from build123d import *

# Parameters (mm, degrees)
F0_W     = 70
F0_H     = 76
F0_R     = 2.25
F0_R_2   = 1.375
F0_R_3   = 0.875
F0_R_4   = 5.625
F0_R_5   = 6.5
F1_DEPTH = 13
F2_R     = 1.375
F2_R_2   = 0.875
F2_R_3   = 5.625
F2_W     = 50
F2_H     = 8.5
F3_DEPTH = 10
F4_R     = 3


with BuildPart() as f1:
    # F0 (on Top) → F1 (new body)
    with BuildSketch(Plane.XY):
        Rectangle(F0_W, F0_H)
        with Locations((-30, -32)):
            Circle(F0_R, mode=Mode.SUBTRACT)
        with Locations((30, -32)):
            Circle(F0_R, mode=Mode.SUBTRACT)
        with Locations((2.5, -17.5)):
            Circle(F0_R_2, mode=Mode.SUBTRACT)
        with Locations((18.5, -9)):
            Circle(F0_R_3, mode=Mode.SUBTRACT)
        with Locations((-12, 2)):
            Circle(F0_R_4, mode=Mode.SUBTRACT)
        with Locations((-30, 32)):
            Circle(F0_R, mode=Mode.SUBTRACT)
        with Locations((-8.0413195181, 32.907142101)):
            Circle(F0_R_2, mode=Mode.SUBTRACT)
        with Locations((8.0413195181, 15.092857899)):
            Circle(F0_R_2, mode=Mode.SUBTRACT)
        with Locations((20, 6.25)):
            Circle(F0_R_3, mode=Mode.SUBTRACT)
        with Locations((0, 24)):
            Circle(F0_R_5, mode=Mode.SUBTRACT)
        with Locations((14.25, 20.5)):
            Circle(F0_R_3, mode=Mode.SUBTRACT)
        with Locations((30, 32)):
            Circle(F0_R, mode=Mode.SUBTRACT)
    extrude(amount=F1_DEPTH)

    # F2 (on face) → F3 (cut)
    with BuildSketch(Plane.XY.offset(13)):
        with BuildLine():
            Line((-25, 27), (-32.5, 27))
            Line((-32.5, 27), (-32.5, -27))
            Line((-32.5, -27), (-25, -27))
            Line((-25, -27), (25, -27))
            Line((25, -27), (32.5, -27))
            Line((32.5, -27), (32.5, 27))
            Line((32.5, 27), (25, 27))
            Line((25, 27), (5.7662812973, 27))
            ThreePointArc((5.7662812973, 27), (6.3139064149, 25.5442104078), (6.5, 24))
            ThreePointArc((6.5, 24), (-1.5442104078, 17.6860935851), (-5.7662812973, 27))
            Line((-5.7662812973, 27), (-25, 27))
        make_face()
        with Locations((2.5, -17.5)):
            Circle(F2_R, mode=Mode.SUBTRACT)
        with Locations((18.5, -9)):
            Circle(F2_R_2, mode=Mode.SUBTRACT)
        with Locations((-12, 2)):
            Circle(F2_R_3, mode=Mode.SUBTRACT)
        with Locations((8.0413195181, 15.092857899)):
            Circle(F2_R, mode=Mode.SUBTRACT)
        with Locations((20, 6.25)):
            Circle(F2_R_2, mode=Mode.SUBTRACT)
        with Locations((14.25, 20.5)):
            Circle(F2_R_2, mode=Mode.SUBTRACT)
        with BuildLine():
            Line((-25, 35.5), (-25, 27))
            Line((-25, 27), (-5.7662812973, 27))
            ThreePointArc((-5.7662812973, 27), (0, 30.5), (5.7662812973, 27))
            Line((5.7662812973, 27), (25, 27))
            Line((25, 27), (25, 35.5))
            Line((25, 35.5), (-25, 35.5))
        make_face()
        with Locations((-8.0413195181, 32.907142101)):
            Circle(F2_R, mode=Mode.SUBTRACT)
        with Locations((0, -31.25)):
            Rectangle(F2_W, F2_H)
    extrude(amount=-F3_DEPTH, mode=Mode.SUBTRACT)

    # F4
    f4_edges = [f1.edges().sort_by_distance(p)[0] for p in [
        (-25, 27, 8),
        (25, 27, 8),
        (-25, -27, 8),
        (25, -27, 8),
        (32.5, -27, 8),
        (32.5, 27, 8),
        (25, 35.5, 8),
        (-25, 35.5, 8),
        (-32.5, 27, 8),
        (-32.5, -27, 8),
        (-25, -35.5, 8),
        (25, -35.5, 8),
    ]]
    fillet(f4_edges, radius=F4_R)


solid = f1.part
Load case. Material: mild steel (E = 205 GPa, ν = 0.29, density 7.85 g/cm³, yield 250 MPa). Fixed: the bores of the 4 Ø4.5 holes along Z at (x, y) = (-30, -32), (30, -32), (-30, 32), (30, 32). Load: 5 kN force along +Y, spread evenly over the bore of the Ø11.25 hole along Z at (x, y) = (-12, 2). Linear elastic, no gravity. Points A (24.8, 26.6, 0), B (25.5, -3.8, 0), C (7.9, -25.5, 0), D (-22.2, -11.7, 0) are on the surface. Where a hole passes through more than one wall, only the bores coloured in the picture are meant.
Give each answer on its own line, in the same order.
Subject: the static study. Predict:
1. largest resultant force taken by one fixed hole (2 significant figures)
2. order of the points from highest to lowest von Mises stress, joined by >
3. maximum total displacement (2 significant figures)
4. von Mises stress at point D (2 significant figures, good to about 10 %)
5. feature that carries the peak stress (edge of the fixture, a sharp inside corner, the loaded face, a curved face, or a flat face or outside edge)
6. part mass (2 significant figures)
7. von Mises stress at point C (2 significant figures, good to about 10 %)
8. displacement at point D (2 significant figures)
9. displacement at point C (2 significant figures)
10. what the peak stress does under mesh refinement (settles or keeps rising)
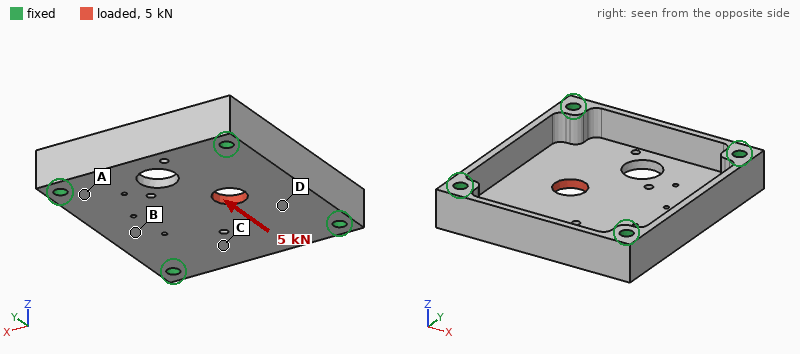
1.8 kN
D > A > C > B
6.8 µm
30 MPa
edge of the fixture
190 g
12 MPa
3.0 µm
2.8 µm
keeps rising
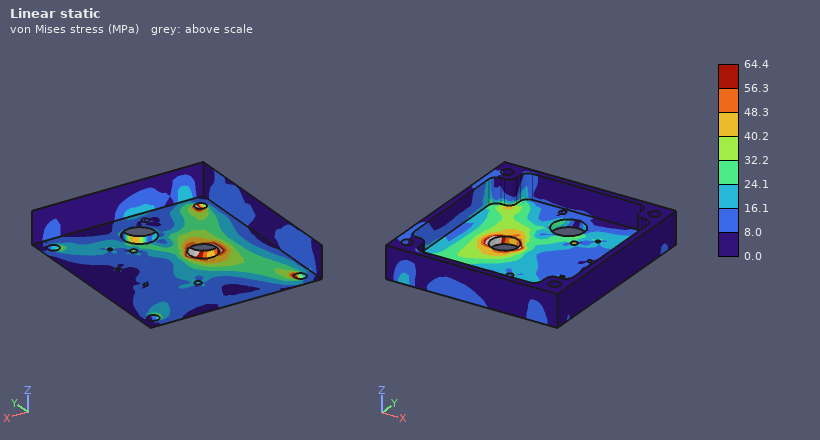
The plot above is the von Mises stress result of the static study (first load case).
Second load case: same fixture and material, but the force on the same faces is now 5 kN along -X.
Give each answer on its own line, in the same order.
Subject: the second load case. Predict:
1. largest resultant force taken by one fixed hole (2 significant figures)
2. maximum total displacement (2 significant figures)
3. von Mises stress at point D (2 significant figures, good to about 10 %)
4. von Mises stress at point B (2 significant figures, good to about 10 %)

1.5 kN
9.6 µm
30 MPa
7.8 MPa
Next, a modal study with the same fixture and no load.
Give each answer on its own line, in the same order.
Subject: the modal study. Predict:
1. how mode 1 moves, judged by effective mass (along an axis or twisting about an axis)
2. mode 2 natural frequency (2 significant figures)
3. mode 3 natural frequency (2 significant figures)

along Z
7800 Hz
8000 Hz
